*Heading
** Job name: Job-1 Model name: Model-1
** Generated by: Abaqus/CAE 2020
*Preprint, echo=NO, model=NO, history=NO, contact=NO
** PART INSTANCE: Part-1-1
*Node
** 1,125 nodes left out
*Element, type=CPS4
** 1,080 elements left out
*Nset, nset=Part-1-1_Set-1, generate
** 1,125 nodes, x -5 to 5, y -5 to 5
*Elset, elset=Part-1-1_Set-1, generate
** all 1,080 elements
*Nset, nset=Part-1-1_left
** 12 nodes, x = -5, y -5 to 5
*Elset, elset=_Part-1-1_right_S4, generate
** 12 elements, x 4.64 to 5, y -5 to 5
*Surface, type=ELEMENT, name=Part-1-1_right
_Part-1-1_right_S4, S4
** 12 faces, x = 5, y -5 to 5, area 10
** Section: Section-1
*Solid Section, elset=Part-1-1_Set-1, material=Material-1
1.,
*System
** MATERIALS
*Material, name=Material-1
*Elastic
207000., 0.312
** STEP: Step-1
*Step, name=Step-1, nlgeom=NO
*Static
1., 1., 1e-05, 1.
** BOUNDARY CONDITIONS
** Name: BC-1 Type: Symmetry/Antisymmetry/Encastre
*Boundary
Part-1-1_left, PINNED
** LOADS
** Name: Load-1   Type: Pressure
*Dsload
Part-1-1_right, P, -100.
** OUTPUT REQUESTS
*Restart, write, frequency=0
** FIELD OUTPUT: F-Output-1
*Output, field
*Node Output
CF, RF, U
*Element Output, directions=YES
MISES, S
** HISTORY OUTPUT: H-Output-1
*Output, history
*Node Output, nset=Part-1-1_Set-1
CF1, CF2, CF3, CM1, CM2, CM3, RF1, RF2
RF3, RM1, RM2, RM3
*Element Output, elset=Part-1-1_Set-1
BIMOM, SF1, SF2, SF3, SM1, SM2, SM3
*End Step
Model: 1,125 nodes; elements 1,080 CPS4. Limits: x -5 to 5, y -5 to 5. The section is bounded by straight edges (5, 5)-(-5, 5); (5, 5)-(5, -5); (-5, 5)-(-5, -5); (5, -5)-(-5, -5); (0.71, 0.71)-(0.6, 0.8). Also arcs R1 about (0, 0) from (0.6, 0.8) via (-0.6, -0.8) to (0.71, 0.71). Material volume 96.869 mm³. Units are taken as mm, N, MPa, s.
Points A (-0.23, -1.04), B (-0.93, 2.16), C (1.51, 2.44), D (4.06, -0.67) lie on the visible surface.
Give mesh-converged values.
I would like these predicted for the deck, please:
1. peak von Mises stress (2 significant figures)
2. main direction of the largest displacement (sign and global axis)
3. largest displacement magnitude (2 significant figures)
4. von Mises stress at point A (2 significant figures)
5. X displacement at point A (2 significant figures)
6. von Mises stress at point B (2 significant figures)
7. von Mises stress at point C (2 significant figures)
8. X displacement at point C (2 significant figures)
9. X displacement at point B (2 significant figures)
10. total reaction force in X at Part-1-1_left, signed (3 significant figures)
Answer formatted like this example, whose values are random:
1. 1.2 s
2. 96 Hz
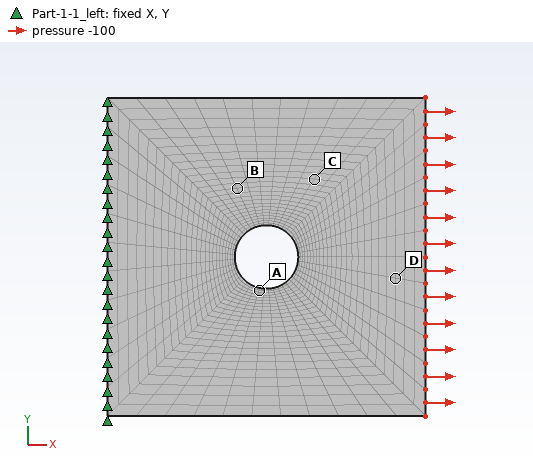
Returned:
1. 320 MPa
2. +X
3. 0.0055 mm
4. 250 MPa
5. 0.0023 mm
6. 130 MPa
7. 120 MPa
8. 0.0035 mm
9. 0.0021 mm
10. -1000 N
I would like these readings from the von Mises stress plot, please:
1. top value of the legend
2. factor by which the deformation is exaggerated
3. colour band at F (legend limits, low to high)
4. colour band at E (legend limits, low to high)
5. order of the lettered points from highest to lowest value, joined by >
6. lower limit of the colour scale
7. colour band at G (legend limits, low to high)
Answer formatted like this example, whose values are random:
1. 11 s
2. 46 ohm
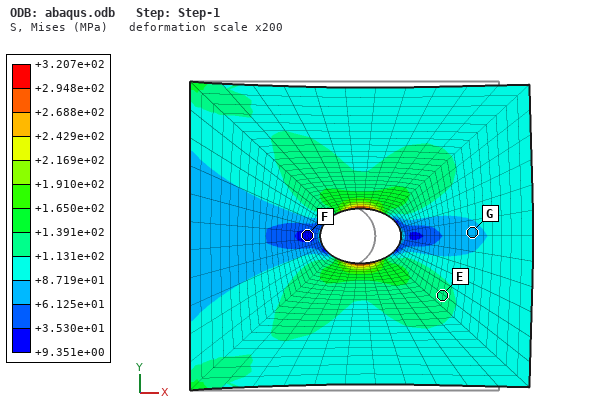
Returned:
1. +3.207e+02 MPa
2. 200
3. +9.351e+00 to +3.530e+01 MPa
4. +1.131e+02 to +1.391e+02 MPa
5. E > G > F
6. +9.351e+00 MPa
7. +6.125e+01 to +8.719e+01 MPa
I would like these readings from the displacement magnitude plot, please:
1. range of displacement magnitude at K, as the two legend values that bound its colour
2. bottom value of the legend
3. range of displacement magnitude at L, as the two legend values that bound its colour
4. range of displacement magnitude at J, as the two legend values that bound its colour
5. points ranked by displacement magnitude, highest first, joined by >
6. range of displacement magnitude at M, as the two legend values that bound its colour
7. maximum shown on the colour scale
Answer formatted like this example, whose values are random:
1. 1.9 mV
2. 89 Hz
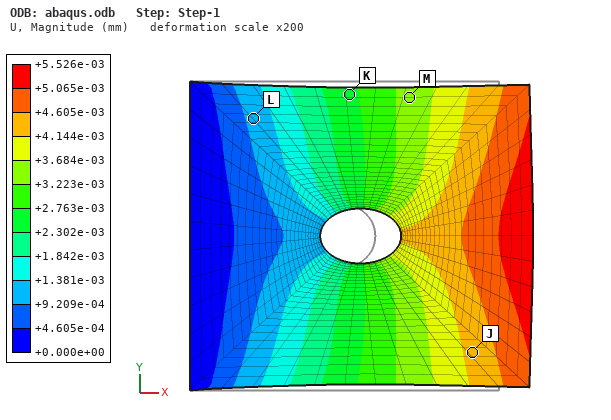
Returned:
1. +2.302e-03 to +2.763e-03 mm
2. +0.000e+00 mm
3. +9.209e-04 to +1.381e-03 mm
4. +4.144e-03 to +4.605e-03 mm
5. J > M > K > L
6. +3.223e-03 to +3.684e-03 mm
7. +5.526e-03 mm
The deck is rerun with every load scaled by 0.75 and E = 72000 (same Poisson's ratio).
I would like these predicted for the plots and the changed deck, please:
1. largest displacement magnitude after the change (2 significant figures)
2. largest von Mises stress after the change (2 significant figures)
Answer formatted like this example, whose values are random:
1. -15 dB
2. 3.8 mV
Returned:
1. 0.012 mm
2. 240 MPa
